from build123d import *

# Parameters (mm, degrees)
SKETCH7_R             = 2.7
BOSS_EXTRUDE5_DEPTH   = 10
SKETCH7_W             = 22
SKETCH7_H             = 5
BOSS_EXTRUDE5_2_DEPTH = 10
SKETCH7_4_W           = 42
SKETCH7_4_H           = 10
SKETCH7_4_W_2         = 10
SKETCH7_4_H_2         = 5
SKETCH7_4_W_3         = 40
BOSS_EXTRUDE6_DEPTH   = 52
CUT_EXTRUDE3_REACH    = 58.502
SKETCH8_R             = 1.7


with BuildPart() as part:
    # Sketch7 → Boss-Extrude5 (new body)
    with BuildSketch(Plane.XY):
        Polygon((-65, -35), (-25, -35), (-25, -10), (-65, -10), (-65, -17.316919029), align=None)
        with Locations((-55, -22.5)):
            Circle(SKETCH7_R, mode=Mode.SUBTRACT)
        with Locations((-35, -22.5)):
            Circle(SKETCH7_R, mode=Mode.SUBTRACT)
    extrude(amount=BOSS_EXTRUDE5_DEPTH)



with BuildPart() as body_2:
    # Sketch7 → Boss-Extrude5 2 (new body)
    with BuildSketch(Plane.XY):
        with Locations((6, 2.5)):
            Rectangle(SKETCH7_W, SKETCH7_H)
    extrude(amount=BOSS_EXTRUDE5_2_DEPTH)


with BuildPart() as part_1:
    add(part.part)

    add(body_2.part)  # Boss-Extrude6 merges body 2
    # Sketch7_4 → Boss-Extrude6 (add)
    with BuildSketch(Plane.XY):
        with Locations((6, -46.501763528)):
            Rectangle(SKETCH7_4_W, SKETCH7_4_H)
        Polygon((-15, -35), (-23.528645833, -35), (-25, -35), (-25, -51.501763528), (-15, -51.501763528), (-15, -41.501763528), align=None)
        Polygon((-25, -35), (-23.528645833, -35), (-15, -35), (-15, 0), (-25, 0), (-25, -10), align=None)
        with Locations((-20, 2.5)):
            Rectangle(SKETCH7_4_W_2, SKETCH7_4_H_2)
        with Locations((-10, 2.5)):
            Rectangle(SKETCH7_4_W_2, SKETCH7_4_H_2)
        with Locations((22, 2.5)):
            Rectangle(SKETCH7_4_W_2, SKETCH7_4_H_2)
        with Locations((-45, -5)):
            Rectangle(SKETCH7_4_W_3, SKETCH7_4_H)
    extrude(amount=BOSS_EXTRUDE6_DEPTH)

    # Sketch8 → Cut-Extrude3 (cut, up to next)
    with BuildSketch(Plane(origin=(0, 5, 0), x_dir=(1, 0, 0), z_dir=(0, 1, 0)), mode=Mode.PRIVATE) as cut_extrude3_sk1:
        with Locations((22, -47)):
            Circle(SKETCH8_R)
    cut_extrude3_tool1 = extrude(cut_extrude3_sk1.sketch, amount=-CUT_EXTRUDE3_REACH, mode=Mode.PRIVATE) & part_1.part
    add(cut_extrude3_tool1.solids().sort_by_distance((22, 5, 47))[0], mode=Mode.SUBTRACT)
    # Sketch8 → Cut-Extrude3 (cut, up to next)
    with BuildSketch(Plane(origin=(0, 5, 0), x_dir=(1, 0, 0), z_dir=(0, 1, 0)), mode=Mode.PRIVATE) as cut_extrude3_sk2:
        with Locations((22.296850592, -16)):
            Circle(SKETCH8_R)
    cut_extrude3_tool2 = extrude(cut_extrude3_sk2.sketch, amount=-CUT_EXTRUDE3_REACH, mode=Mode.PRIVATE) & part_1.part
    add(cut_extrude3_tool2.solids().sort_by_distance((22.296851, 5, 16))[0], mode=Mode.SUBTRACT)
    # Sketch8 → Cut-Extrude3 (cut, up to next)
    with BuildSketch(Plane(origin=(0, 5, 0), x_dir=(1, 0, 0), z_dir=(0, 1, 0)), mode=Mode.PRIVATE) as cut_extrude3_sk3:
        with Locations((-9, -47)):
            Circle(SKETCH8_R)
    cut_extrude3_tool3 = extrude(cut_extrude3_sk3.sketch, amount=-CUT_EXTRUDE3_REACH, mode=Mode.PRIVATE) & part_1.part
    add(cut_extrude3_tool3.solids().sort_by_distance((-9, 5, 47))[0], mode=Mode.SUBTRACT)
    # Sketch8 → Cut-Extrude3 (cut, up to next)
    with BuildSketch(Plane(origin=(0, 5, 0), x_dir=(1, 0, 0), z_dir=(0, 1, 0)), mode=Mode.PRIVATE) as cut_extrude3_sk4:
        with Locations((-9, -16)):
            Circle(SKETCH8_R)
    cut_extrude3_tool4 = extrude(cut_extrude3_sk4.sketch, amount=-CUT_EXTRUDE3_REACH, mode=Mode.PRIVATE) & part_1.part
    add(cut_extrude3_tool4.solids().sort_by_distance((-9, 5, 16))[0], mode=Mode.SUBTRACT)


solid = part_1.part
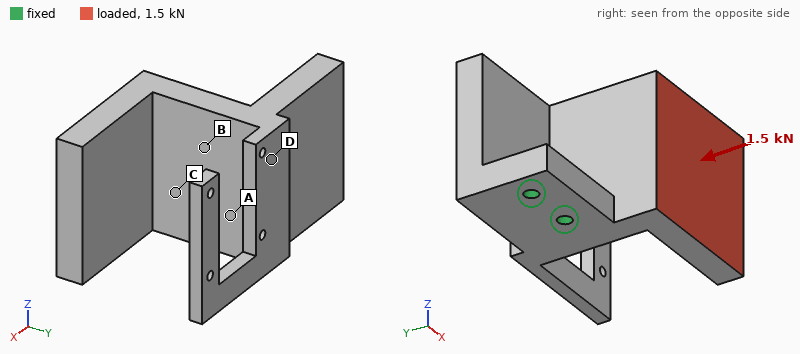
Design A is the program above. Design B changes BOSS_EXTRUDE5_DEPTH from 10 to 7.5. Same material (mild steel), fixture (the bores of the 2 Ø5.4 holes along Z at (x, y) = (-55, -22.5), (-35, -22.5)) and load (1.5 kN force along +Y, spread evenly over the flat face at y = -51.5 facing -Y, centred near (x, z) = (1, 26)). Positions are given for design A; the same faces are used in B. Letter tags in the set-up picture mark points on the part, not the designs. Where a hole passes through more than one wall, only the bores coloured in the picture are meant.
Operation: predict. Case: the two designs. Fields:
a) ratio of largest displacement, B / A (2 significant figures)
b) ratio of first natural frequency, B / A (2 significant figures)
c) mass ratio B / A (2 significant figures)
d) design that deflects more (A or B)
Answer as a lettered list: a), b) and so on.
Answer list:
a) 1.3
b) 0.99
c) 0.97
d) B
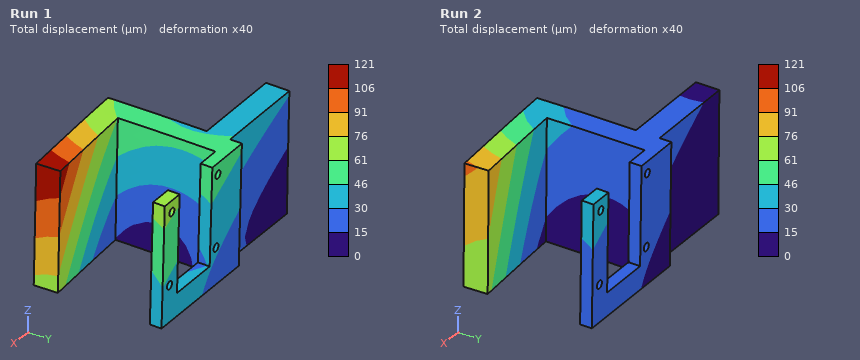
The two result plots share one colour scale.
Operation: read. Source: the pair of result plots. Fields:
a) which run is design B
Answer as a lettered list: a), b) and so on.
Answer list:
a) Run 1
